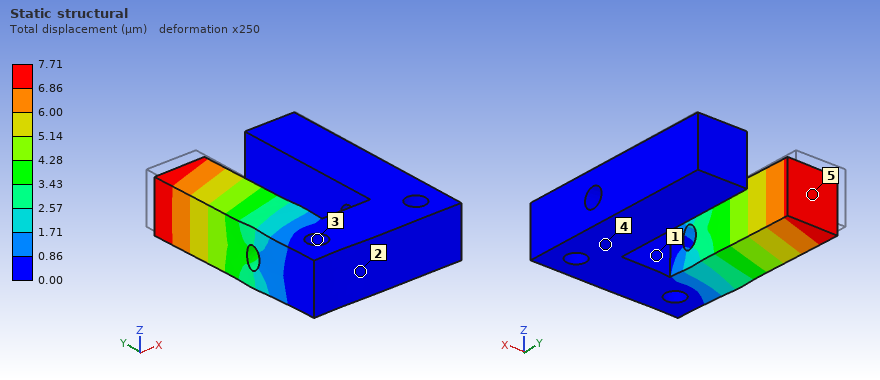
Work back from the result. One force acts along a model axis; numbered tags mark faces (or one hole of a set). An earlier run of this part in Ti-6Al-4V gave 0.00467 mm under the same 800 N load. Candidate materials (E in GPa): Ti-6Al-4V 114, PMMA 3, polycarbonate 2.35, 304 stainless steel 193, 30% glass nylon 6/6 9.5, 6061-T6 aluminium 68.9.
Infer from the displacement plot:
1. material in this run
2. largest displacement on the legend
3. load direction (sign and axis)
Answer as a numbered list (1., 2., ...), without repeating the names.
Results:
1. 6061-T6 aluminium
2. 7.71 µm
3. -Y
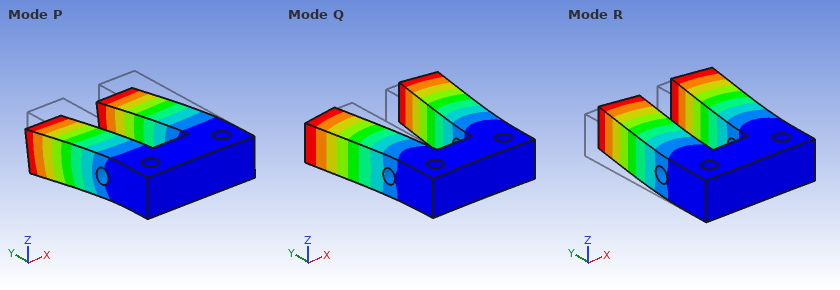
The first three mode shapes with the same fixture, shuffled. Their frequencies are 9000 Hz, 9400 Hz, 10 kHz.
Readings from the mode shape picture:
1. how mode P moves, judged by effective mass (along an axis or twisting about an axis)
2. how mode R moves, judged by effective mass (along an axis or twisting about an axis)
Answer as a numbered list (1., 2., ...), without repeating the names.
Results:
1. along Z
2. along X
